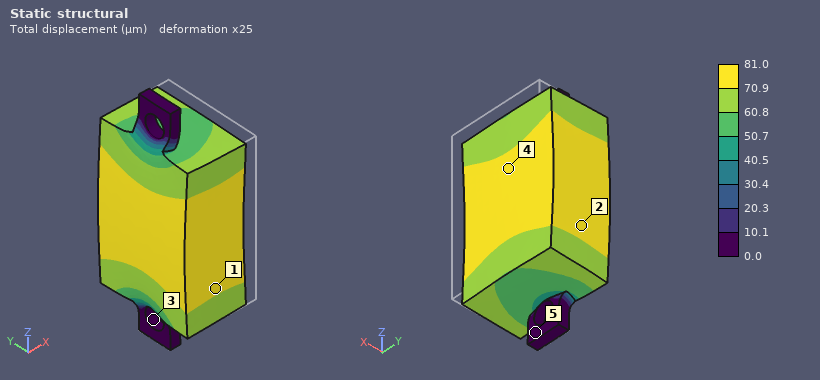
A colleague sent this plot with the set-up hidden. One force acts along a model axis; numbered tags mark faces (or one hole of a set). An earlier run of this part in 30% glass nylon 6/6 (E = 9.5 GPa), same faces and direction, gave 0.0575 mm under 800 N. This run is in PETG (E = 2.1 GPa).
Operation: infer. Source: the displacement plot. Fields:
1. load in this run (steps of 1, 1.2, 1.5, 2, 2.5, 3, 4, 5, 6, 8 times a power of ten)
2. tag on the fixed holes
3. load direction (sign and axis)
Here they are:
250 N
3
-X
